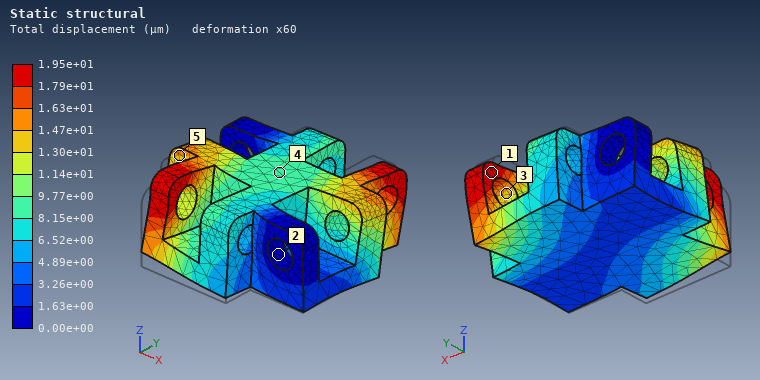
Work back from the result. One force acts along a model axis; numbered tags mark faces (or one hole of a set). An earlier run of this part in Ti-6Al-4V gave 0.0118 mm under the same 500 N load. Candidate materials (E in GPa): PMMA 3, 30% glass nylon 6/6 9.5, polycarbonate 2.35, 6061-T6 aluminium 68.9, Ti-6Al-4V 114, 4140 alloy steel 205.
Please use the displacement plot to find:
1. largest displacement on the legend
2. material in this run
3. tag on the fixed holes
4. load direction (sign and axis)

1.95e+01 µm
6061-T6 aluminium
2
+Y
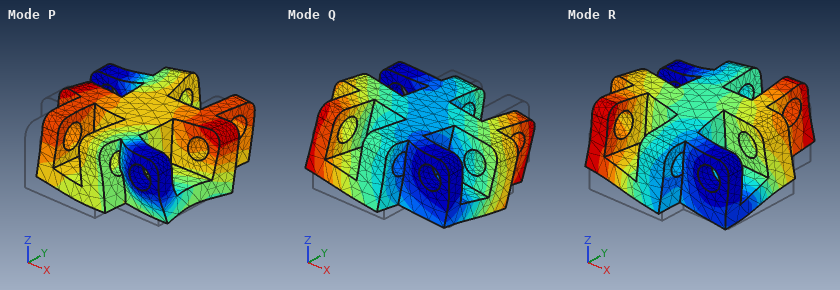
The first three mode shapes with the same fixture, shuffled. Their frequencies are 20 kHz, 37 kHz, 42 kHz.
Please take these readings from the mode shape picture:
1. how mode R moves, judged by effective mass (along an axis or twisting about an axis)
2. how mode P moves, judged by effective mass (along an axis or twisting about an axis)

along Z
along Y
